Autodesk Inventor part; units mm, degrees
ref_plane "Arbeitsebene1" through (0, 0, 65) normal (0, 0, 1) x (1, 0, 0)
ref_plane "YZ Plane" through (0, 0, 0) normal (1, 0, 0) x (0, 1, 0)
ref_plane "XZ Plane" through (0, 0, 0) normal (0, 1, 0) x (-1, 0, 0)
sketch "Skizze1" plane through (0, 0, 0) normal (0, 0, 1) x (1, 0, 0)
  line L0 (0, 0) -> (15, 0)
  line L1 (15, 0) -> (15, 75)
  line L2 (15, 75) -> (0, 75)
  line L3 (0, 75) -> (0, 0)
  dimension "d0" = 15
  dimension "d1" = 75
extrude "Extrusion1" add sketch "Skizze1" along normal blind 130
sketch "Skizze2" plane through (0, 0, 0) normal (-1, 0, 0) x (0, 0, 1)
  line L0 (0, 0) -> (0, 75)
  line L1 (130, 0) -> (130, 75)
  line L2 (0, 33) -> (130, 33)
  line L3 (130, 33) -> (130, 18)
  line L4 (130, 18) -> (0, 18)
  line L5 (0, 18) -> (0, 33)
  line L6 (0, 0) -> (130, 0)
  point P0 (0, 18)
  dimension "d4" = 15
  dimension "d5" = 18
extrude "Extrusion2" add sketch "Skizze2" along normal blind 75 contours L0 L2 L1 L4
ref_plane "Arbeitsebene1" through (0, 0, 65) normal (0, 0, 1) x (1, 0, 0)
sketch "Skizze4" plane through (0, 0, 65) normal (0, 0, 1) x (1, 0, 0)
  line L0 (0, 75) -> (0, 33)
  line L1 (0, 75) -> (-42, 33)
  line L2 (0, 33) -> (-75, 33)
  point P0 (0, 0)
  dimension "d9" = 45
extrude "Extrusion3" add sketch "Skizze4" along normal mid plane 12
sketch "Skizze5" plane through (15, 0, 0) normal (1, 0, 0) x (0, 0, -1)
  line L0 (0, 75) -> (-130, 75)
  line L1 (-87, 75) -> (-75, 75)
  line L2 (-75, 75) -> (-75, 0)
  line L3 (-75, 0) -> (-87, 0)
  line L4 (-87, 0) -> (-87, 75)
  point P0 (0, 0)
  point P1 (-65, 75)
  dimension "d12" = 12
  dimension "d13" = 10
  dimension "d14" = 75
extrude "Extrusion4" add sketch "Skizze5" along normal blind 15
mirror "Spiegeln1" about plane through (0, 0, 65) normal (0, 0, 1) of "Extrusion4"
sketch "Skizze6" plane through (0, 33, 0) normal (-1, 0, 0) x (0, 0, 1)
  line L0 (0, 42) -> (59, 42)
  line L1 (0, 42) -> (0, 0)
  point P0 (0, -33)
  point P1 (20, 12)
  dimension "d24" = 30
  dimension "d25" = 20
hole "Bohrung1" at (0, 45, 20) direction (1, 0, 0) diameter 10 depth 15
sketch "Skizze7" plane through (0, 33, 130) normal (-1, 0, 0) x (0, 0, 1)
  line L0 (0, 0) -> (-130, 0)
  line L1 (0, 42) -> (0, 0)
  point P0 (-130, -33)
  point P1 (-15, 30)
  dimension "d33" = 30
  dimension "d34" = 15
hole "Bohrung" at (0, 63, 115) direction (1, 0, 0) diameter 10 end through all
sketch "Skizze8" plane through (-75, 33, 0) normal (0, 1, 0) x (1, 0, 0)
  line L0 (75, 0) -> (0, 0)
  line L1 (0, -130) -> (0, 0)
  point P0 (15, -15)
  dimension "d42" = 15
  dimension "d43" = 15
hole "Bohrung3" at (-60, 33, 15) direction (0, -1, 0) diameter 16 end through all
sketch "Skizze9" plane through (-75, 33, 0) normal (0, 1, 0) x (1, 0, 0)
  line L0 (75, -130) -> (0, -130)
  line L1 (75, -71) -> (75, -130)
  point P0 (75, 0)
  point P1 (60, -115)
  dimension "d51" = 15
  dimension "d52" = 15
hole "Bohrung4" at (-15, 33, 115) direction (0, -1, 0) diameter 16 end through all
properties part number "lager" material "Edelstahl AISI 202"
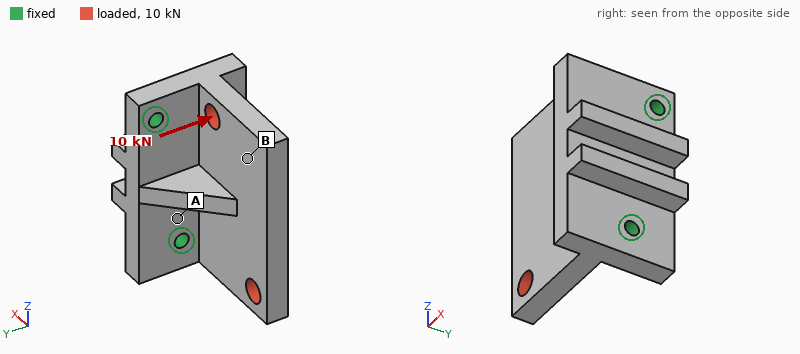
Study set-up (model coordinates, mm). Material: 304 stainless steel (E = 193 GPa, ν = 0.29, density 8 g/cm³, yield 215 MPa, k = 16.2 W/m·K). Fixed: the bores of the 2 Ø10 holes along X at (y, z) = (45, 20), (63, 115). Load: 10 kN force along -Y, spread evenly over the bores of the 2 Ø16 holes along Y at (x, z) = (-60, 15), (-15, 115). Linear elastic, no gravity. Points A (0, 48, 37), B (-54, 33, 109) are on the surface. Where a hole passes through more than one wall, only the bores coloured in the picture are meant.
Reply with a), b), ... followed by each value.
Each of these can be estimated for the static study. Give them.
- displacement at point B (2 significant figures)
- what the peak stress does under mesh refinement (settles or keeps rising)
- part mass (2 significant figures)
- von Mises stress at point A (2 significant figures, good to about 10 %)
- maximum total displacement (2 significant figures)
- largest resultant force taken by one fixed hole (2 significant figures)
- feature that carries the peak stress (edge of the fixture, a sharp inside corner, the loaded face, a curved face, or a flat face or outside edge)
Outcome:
a) 0.10 mm
b) keeps rising
c) 2.6 kg
d) 52 MPa
e) 0.24 mm
f) 5.3 kN
g) edge of the fixture
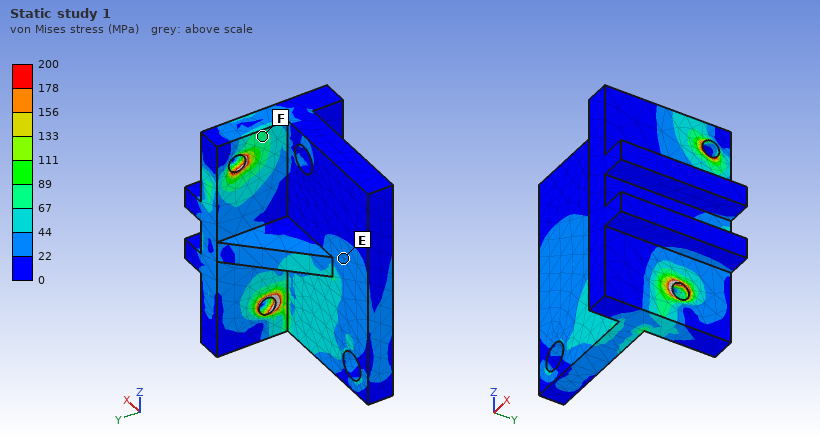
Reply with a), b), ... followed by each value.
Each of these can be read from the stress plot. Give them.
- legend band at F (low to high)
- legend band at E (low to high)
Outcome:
a) 67 to 89 MPa
b) 22 to 44 MPa
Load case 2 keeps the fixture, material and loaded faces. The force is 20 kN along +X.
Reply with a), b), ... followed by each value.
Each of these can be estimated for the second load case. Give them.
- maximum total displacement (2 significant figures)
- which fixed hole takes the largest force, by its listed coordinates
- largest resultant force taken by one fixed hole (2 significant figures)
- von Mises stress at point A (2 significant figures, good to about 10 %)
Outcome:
a) 0.14 mm
b) (45, 20)
c) 11 kN
d) 44 MPa
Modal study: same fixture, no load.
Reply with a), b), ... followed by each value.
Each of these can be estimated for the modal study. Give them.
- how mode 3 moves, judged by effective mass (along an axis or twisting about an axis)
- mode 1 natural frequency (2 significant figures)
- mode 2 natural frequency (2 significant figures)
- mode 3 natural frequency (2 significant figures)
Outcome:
a) along X
b) 1300 Hz
c) 2600 Hz
d) 3000 Hz
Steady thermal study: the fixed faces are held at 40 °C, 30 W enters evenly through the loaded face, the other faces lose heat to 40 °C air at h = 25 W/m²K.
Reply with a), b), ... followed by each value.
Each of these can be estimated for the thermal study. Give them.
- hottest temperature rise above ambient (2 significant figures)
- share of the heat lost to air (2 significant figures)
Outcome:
a) 61 K
b) 66 %
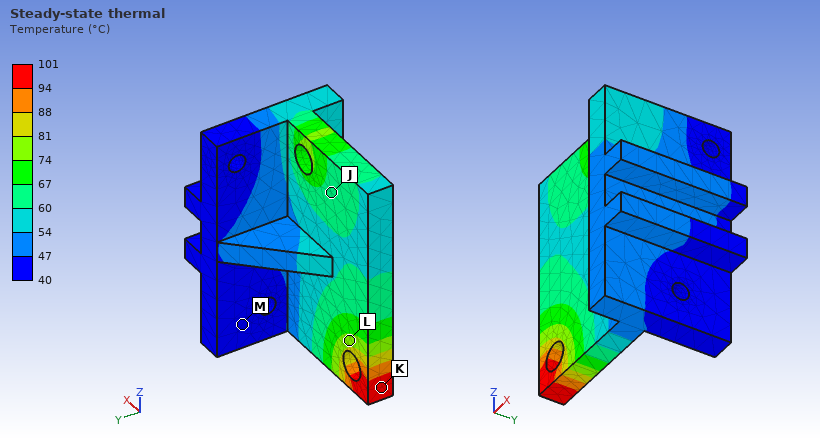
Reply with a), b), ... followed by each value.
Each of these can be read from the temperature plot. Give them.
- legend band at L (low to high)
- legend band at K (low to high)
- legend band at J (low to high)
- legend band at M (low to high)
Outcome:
a) 74 to 81 °C
b) 94 to 101 °C
c) 60 to 67 °C
d) 40 to 47 °C
